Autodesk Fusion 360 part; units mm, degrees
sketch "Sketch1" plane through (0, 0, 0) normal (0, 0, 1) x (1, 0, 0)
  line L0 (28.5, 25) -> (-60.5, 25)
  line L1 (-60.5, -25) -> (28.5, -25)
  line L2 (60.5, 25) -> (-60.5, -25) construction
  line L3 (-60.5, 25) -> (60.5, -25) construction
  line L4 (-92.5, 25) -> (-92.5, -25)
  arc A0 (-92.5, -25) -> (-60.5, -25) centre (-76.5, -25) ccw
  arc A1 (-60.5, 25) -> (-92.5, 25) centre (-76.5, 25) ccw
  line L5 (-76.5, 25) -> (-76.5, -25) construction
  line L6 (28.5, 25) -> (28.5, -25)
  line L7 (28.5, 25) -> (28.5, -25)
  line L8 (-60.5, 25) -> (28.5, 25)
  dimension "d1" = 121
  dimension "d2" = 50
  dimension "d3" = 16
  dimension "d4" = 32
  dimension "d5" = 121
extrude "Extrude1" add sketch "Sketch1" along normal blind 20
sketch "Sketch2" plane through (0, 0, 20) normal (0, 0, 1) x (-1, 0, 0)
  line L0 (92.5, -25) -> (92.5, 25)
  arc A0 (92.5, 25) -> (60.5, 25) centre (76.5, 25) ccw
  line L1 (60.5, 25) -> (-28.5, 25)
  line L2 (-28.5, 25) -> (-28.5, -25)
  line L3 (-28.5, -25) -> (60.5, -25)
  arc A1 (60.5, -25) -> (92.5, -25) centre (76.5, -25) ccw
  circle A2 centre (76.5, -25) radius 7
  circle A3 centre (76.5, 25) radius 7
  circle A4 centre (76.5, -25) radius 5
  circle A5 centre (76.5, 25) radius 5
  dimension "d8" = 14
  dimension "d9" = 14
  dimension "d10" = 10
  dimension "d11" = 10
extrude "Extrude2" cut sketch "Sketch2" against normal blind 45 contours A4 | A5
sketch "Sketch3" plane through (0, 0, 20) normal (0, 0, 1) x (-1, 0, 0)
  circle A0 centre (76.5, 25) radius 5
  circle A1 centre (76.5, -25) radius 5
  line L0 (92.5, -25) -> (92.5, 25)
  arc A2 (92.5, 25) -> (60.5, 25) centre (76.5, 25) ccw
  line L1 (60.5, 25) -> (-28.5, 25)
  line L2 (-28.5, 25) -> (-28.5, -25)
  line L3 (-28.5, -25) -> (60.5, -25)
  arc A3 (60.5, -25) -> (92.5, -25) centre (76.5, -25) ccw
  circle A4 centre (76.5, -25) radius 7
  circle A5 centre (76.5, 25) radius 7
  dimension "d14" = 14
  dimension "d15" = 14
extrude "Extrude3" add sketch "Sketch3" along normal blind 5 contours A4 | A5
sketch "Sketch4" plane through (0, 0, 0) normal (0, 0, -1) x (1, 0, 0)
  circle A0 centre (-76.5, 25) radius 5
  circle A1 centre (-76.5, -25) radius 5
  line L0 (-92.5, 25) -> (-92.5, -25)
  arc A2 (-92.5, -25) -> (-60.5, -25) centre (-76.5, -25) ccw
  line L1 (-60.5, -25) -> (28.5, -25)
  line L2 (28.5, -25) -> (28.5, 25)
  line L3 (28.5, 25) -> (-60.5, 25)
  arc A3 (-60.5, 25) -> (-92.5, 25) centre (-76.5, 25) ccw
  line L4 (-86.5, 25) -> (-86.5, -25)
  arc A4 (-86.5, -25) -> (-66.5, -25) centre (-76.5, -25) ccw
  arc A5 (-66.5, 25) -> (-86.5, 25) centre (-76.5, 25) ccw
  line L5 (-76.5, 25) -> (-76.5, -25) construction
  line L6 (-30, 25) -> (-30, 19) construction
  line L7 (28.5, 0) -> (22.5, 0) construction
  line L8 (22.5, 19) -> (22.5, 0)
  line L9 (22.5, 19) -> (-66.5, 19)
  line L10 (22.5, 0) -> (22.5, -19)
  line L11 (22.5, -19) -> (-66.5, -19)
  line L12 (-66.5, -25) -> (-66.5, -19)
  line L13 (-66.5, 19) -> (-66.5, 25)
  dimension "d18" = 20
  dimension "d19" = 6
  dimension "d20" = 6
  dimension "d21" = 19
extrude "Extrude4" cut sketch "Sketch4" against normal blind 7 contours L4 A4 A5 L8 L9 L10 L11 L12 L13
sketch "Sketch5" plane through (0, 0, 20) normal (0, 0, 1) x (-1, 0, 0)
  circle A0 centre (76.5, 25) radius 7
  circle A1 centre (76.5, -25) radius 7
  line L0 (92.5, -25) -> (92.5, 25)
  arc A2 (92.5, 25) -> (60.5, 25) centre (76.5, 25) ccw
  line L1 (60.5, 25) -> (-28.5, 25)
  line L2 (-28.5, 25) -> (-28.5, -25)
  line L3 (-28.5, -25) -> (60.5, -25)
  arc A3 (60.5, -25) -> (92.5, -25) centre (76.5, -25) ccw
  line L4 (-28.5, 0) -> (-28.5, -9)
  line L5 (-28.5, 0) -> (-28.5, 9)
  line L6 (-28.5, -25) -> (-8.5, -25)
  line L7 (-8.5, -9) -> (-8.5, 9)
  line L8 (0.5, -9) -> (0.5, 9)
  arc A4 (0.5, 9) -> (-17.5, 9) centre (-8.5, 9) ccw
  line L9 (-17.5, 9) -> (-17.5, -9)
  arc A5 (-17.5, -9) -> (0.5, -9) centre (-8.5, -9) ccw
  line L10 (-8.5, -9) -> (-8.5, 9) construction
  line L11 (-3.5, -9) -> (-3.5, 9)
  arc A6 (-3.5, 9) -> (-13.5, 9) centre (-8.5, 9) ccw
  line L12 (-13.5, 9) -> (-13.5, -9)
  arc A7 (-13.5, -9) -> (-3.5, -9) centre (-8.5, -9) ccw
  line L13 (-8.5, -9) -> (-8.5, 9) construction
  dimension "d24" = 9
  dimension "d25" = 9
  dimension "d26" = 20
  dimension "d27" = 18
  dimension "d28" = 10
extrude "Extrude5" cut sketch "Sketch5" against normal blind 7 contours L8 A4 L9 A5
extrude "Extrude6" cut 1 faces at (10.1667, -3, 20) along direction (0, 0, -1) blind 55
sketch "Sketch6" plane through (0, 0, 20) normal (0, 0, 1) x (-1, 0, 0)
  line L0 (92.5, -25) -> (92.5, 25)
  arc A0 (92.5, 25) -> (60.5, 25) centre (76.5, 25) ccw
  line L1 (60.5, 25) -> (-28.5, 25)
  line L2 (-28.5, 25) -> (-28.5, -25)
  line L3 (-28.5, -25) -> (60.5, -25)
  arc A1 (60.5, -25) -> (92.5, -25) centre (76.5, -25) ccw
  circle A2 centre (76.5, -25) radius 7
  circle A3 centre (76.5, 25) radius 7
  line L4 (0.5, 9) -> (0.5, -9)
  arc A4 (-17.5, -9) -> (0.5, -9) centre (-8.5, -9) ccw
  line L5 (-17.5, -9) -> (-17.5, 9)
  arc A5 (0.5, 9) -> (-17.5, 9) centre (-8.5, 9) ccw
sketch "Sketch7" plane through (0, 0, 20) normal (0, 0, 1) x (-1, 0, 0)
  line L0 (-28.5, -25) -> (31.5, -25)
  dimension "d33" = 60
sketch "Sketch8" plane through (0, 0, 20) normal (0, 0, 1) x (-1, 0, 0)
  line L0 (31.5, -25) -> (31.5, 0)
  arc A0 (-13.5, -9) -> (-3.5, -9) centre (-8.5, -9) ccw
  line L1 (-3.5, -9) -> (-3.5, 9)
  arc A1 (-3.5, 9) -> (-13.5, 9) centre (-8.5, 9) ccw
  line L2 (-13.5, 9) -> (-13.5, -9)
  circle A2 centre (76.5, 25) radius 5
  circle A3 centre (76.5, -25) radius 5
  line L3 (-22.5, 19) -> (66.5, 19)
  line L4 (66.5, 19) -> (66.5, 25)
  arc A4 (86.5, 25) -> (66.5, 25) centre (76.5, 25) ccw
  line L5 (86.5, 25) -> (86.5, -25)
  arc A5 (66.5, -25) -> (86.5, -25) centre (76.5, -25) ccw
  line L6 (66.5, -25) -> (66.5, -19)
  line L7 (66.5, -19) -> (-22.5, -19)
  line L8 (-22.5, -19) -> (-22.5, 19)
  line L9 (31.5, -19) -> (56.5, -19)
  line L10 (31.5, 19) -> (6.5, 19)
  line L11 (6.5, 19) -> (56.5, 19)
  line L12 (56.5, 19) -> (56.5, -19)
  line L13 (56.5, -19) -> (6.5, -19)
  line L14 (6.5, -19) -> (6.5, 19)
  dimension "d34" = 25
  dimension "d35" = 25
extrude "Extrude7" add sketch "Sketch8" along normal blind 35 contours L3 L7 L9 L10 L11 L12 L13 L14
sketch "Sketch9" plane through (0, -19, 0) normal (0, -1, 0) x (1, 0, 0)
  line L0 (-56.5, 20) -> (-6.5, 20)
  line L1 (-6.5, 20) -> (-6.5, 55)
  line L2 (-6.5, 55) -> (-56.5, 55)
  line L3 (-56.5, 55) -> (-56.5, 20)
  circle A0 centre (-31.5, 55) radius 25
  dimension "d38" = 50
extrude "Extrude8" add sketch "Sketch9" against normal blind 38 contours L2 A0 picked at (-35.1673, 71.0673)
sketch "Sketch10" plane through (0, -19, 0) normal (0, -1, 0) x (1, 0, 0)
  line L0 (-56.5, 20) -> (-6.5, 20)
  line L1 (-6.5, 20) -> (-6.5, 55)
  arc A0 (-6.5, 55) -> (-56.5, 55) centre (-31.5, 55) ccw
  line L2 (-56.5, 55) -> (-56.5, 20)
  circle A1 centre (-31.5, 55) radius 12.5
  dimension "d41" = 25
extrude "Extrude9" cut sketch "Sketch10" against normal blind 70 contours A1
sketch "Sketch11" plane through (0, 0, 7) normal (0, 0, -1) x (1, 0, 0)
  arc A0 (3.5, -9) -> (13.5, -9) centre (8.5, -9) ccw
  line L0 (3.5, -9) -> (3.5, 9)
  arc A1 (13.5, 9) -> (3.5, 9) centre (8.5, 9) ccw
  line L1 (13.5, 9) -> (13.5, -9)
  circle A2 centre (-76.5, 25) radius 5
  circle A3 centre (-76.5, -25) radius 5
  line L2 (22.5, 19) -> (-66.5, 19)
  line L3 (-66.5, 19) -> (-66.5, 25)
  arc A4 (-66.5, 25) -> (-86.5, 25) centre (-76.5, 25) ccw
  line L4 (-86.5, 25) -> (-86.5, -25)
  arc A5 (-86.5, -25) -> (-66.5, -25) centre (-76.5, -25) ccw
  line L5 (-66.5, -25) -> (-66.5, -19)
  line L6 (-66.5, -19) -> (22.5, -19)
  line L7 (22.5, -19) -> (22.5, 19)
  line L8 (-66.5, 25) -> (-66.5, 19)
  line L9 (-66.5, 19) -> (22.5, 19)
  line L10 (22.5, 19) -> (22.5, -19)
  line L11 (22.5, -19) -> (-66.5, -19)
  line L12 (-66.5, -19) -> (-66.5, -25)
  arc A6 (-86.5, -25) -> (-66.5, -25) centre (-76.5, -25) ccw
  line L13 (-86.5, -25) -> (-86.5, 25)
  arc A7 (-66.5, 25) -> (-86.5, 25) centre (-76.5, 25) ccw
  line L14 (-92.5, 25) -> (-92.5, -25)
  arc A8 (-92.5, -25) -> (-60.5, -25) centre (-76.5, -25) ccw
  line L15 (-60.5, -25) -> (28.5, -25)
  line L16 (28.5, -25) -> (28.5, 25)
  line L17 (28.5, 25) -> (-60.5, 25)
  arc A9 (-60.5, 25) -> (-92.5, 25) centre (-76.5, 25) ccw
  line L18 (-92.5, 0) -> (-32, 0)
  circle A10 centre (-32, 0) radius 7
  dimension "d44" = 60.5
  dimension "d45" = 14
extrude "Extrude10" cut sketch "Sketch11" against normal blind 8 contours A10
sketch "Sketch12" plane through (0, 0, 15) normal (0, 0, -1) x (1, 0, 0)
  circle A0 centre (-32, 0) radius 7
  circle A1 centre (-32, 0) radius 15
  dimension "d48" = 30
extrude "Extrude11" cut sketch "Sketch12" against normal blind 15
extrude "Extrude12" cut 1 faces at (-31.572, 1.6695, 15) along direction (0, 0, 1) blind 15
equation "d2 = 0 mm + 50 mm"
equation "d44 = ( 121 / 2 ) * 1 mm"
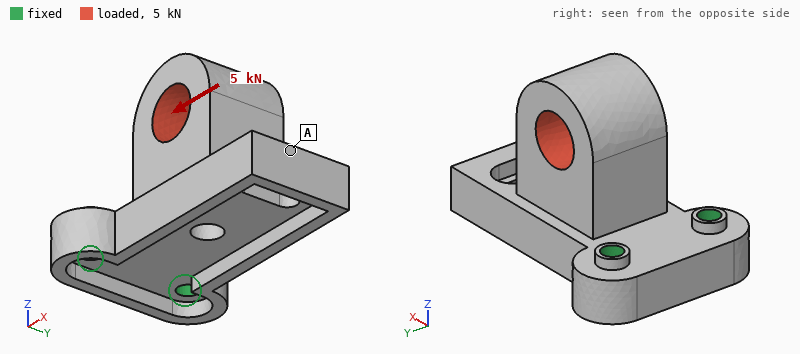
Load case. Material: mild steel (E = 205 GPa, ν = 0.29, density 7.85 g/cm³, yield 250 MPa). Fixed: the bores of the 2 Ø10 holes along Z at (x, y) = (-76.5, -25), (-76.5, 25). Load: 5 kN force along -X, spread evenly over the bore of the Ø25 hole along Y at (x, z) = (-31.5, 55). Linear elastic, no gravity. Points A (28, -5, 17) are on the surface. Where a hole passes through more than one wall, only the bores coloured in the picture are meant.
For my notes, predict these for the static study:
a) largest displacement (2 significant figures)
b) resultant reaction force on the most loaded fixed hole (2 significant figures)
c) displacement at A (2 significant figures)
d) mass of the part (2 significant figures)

0.20 mm
2.6 kN
0.20 mm
1.3 kg
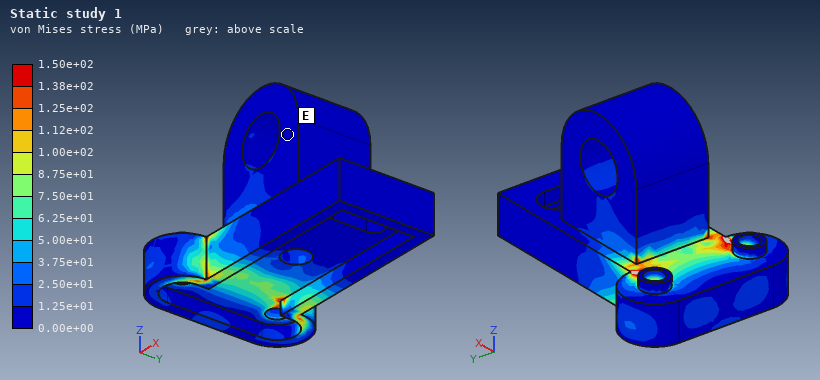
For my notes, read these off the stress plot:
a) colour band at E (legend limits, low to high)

0.00e+00 to 1.25e+01 MPa
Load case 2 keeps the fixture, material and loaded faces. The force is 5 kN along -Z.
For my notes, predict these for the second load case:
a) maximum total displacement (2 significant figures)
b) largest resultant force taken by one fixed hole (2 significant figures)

0.16 mm
2.5 kN
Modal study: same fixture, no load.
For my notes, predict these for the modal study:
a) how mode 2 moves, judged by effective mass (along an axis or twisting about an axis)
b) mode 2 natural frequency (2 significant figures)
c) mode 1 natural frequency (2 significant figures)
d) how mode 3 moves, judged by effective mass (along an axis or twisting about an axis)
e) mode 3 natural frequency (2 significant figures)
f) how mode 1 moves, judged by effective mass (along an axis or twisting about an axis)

along Y
2300 Hz
880 Hz
along Y
3300 Hz
along Z
